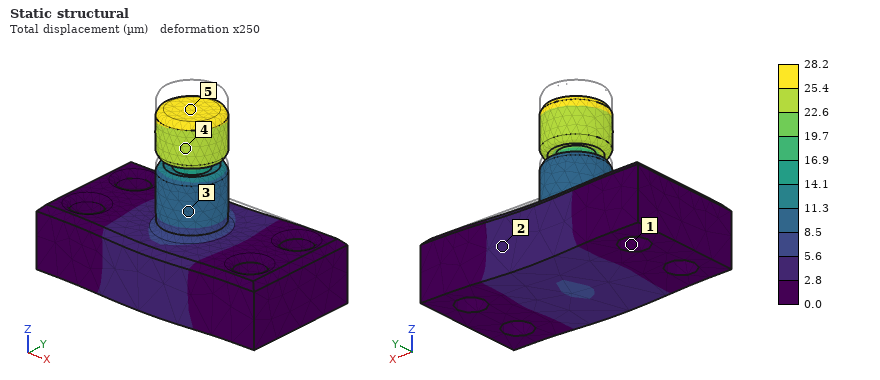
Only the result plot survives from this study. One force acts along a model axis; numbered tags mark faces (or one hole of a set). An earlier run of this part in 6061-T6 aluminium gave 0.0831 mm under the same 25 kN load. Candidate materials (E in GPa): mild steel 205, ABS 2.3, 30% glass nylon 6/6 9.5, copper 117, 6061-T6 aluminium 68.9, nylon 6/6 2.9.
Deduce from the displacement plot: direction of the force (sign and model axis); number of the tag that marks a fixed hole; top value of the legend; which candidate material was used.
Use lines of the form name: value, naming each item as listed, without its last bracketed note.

direction of the force: -Z
number of the tag that marks a fixed hole: 1
top value of the legend: 28.2 µm
which candidate material was used: mild steel
